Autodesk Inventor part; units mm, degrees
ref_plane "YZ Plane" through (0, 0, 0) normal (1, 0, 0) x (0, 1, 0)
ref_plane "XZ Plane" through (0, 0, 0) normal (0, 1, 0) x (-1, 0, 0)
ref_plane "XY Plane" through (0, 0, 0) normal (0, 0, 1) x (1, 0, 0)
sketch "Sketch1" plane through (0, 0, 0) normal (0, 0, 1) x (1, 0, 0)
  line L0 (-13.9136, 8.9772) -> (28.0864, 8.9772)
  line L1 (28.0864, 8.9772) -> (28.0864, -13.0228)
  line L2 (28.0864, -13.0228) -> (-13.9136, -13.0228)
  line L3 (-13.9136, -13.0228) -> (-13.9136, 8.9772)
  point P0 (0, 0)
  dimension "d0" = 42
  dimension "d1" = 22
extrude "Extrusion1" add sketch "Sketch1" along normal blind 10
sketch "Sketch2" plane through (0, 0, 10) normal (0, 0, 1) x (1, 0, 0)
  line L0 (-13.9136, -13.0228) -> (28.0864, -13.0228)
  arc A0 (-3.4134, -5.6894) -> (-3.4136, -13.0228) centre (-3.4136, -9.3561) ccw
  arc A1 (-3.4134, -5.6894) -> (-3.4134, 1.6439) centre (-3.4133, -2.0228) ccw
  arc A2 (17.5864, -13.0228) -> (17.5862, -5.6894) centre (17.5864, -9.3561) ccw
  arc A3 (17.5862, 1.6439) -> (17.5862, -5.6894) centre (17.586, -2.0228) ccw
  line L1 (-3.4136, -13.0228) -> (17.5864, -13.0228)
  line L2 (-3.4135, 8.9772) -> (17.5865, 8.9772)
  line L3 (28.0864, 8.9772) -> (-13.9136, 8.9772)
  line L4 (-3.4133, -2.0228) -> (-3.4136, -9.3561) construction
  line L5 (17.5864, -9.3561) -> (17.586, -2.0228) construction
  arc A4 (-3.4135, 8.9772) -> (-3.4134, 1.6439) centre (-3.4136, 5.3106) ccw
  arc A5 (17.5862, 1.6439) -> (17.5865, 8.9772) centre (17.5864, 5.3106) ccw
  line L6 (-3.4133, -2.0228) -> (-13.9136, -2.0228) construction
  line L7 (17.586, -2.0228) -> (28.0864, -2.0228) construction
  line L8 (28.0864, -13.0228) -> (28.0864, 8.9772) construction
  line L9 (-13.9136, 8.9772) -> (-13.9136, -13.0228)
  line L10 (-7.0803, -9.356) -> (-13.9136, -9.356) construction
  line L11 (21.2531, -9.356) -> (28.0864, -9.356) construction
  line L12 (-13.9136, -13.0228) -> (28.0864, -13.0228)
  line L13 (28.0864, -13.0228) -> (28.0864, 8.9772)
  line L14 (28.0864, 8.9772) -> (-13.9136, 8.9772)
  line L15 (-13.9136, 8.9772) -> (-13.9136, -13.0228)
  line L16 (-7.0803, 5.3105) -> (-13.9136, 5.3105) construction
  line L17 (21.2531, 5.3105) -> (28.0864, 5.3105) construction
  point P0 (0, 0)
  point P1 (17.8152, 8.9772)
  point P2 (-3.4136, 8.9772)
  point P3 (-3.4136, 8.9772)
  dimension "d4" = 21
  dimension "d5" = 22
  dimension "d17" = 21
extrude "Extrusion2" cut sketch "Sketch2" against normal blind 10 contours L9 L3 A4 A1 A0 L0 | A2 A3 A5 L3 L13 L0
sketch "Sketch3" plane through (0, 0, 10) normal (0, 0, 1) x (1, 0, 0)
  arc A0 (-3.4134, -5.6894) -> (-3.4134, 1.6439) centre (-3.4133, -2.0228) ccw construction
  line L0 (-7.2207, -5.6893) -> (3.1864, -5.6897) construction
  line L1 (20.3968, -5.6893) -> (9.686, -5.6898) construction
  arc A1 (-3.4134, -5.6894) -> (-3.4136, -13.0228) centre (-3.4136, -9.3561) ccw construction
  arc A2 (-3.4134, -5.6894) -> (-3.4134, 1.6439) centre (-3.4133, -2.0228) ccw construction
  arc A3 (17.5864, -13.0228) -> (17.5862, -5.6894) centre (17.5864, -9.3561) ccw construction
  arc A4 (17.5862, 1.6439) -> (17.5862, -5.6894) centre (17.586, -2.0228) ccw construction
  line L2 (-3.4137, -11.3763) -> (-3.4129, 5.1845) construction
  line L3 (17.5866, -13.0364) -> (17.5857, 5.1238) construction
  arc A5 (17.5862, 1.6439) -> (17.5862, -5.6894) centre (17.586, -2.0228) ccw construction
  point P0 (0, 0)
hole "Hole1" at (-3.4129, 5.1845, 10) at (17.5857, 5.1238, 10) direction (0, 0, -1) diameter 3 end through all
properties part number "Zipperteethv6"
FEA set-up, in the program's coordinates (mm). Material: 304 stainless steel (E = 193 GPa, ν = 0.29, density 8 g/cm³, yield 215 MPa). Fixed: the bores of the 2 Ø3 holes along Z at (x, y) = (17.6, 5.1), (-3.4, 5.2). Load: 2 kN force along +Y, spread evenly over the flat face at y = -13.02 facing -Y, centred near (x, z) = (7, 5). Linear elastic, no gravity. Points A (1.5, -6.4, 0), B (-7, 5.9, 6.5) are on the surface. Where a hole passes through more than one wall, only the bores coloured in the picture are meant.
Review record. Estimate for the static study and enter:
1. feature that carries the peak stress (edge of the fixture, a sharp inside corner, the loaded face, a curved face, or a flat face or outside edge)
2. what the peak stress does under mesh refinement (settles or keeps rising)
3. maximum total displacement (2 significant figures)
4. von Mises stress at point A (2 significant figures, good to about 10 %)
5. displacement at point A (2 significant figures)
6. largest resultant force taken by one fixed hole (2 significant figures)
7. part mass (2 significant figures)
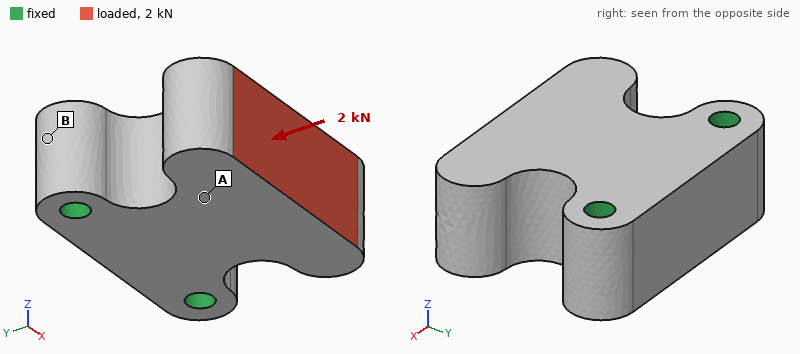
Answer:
edge of the fixture
keeps rising
2.4 µm
14 MPa
1.7 µm
1.1 kN
39 g
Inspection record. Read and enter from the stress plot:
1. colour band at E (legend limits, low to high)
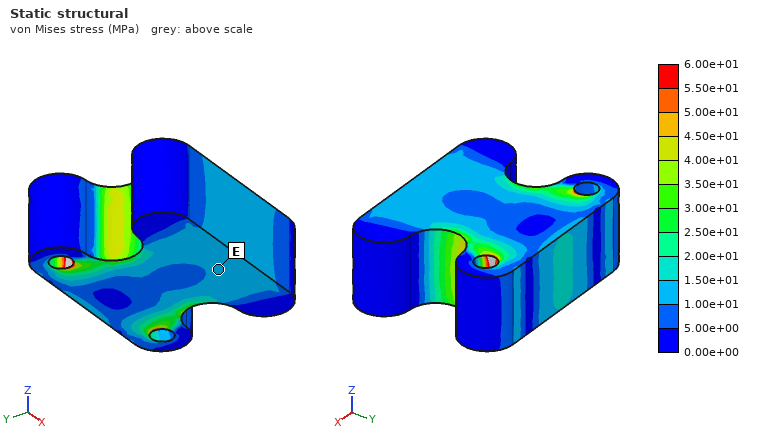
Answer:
1.00e+01 to 1.50e+01 MPa
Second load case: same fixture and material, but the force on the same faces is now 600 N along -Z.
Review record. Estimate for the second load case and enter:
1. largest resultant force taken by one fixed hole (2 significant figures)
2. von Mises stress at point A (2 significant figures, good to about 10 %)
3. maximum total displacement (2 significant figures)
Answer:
300 N
14 MPa
11 µm
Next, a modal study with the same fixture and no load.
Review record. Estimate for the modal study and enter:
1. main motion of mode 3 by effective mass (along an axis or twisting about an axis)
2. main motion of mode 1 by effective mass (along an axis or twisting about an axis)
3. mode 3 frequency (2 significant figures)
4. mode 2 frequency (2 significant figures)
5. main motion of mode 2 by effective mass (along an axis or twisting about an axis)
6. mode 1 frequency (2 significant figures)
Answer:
twisting about Y
along Z
20 kHz
19 kHz
along X
11 kHz
